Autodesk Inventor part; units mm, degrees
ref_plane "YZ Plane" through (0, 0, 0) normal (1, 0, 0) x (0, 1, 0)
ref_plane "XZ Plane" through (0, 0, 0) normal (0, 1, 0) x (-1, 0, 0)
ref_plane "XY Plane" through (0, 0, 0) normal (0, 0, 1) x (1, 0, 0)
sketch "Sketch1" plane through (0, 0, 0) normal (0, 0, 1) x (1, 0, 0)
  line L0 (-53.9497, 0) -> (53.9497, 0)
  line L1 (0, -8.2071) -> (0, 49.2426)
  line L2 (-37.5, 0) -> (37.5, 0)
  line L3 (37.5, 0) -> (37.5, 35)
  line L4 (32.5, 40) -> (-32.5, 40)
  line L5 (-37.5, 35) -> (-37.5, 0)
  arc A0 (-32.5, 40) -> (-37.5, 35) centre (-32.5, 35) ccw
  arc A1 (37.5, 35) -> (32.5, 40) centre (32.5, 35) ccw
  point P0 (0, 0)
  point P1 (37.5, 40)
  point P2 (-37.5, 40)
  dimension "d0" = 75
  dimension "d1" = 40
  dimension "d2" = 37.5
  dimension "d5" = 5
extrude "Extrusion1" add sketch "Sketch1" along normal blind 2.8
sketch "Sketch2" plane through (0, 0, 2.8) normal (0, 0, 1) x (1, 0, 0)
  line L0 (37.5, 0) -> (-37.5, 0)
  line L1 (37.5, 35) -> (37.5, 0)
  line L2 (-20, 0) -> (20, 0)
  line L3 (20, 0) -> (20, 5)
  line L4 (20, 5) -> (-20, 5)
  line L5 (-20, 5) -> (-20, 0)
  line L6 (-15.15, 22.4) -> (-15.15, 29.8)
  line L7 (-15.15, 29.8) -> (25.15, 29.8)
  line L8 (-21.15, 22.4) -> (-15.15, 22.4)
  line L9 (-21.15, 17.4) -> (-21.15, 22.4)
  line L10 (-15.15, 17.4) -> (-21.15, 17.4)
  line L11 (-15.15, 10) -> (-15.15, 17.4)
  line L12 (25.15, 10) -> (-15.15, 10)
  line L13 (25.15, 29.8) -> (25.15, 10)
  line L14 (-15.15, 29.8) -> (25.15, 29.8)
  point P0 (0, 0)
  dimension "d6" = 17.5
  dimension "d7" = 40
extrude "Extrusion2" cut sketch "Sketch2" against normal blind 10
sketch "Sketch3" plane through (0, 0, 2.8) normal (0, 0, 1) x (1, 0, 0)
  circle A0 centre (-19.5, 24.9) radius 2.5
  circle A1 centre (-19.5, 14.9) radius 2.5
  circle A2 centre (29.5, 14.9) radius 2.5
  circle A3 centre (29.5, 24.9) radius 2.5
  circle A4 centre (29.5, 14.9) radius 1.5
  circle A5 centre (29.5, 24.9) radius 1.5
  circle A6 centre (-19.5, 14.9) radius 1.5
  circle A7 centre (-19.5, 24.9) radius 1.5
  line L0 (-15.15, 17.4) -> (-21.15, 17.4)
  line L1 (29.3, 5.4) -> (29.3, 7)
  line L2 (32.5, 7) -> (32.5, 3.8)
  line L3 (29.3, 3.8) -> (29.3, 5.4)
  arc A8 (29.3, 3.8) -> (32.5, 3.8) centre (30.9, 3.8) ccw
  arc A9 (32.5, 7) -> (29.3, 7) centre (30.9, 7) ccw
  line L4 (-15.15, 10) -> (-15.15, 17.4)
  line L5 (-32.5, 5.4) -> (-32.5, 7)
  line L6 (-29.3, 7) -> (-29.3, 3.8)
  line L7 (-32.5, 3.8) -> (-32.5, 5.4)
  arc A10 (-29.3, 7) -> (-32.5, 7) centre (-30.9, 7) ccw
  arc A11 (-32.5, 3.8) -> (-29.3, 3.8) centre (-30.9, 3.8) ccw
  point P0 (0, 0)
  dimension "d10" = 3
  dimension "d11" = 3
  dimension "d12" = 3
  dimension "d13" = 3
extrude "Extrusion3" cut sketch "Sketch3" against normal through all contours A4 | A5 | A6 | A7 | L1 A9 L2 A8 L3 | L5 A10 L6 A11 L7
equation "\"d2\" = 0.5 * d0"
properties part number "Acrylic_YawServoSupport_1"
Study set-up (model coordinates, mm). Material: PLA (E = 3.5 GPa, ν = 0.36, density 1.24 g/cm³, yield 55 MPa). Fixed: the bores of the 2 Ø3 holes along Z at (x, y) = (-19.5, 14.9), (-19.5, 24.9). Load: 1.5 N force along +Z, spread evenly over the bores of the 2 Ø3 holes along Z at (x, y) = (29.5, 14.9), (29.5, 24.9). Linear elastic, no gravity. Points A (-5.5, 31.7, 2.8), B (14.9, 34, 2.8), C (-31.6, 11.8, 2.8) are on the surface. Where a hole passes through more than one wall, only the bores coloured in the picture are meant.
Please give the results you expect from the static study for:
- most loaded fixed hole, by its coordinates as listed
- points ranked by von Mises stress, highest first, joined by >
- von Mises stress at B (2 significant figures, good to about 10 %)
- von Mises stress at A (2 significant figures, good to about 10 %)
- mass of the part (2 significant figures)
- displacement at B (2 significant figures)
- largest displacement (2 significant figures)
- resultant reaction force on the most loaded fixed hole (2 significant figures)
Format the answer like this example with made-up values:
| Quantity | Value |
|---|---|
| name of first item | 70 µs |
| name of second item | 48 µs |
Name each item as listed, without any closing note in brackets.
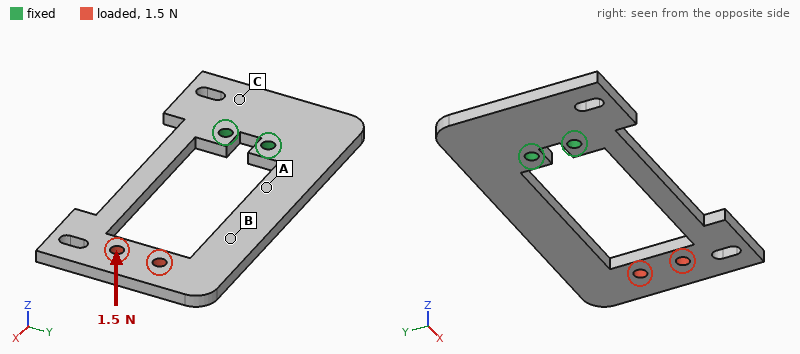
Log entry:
| Quantity | Value |
|---|---|
| most loaded fixed hole, by its coordinates as listed | (-19.5, 14.9) |
| points ranked by von Mises stress, highest first, joined by > | A > B > C |
| von Mises stress at B | 1.2 MPa |
| von Mises stress at A | 2.5 MPa |
| mass of the part | 6.6 g |
| displacement at B | 0.39 mm |
| largest displacement | 0.88 mm |
| resultant reaction force on the most loaded fixed hole | 0.88 N |
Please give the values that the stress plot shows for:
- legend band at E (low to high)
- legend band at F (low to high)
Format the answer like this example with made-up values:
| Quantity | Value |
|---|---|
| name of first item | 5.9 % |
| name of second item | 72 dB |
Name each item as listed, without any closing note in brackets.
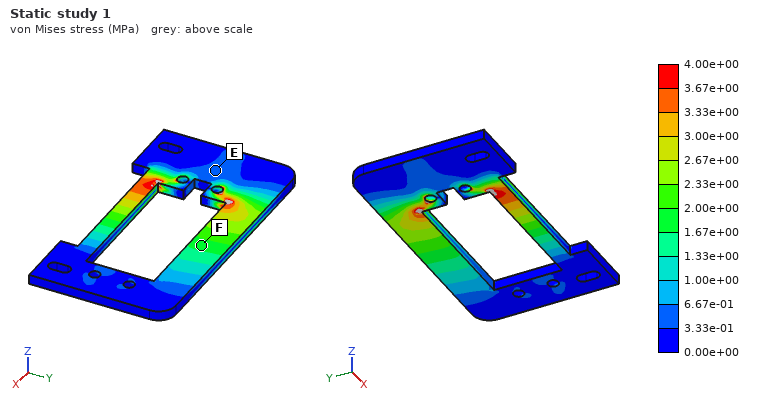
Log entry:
| Quantity | Value |
|---|---|
| legend band at E | 3.33e-01 to 6.67e-01 MPa |
| legend band at F | 1.67e+00 to 2.00e+00 MPa |
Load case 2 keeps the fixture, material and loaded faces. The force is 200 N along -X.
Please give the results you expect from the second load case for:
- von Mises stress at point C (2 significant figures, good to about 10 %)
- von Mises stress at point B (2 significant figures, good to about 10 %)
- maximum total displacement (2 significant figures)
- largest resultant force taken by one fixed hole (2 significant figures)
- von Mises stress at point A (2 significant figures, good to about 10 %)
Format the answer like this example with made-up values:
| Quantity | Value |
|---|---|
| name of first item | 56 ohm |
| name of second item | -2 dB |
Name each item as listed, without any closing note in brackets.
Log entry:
| Quantity | Value |
|---|---|
| von Mises stress at point C | 2.5 MPa |
| von Mises stress at point B | 4.1 MPa |
| maximum total displacement | 0.20 mm |
| largest resultant force taken by one fixed hole | 110 N |
| von Mises stress at point A | 5.3 MPa |
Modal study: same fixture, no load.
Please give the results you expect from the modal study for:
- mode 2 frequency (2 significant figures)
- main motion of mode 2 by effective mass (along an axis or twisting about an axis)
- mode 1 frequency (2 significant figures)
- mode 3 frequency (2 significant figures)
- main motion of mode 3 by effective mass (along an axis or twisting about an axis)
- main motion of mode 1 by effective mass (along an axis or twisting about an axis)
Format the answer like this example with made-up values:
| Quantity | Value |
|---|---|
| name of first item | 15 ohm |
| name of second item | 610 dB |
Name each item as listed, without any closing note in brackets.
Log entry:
| Quantity | Value |
|---|---|
| mode 2 frequency | 460 Hz |
| main motion of mode 2 by effective mass | twisting about X |
| mode 1 frequency | 160 Hz |
| mode 3 frequency | 730 Hz |
| main motion of mode 3 by effective mass | along Y |
| main motion of mode 1 by effective mass | along Z |
